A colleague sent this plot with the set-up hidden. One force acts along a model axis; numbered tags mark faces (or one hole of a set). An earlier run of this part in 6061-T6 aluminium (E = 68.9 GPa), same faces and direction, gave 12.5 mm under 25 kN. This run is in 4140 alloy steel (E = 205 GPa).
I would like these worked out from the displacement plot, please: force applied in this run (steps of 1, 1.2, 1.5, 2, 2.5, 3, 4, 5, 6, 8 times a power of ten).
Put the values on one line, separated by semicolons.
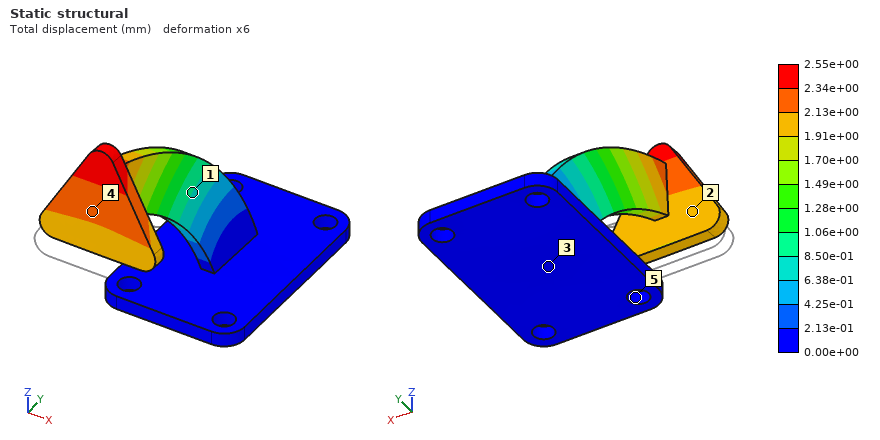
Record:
15 kN
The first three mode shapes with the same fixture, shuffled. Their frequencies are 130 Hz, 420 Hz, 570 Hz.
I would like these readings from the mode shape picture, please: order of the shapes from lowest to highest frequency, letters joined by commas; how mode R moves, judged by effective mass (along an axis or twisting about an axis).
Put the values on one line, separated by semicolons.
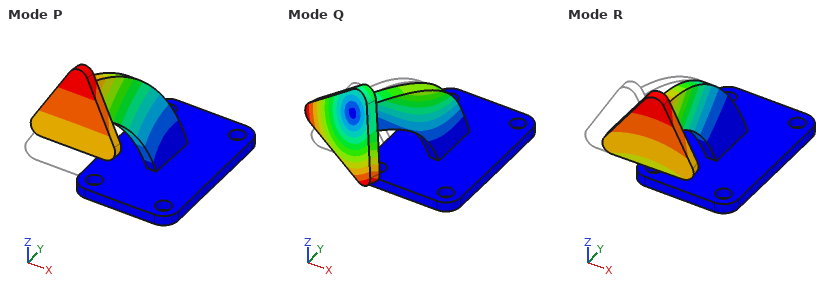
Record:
R, P, Q; along X
